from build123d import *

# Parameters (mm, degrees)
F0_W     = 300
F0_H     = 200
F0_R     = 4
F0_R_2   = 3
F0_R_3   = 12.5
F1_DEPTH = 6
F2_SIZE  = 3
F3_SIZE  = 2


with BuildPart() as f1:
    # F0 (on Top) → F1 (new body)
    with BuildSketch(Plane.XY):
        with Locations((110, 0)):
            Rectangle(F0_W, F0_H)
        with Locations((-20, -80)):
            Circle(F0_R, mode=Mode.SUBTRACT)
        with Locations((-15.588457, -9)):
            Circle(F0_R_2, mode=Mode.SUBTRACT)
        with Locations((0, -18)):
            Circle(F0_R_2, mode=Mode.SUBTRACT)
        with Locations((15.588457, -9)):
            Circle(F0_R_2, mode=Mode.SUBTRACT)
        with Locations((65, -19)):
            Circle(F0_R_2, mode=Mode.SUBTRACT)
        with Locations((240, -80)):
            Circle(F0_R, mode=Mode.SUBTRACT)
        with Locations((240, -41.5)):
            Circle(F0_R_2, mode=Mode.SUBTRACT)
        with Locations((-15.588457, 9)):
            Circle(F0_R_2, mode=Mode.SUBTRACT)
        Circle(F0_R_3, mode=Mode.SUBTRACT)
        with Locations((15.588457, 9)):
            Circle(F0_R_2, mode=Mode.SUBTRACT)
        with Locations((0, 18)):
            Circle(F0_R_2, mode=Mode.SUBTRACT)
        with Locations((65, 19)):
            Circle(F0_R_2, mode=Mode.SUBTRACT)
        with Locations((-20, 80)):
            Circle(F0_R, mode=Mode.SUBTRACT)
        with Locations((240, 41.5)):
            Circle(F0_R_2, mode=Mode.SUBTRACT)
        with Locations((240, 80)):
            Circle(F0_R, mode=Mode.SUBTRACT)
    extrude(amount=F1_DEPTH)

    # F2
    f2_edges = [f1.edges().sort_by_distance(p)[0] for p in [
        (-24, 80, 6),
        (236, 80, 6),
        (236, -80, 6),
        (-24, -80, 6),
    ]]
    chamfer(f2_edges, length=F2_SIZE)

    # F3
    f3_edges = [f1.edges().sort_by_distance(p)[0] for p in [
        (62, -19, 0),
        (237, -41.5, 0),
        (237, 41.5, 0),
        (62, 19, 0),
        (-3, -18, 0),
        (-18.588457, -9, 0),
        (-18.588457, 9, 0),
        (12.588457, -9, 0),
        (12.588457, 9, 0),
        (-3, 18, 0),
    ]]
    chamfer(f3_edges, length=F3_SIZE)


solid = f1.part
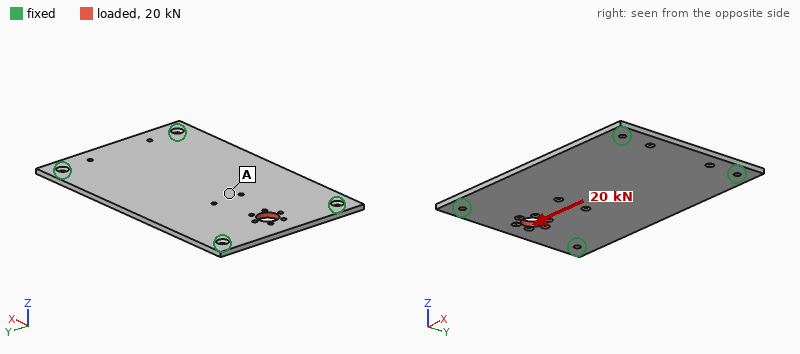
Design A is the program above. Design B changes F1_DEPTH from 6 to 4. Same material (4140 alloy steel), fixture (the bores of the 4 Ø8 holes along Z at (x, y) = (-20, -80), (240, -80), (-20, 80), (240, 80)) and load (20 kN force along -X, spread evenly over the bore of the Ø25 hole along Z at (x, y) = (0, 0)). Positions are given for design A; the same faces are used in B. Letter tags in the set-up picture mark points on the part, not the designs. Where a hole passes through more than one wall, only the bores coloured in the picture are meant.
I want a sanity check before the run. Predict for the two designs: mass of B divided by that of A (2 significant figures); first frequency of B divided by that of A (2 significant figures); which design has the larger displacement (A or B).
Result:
0.67
0.65
B
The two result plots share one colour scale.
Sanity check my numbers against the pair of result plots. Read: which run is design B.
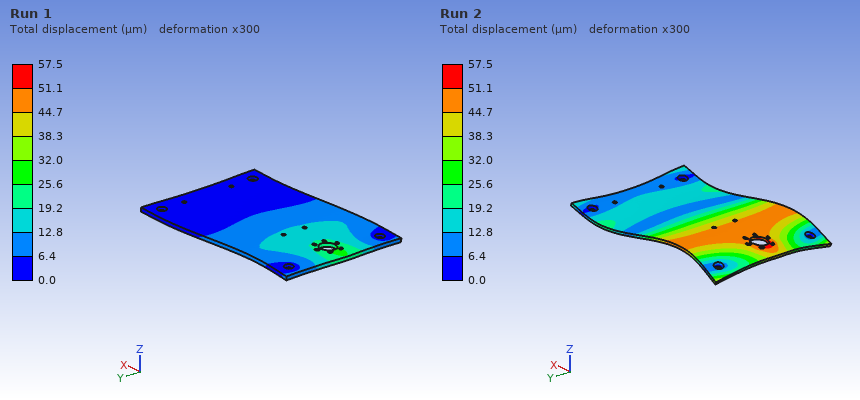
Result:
Run 2
